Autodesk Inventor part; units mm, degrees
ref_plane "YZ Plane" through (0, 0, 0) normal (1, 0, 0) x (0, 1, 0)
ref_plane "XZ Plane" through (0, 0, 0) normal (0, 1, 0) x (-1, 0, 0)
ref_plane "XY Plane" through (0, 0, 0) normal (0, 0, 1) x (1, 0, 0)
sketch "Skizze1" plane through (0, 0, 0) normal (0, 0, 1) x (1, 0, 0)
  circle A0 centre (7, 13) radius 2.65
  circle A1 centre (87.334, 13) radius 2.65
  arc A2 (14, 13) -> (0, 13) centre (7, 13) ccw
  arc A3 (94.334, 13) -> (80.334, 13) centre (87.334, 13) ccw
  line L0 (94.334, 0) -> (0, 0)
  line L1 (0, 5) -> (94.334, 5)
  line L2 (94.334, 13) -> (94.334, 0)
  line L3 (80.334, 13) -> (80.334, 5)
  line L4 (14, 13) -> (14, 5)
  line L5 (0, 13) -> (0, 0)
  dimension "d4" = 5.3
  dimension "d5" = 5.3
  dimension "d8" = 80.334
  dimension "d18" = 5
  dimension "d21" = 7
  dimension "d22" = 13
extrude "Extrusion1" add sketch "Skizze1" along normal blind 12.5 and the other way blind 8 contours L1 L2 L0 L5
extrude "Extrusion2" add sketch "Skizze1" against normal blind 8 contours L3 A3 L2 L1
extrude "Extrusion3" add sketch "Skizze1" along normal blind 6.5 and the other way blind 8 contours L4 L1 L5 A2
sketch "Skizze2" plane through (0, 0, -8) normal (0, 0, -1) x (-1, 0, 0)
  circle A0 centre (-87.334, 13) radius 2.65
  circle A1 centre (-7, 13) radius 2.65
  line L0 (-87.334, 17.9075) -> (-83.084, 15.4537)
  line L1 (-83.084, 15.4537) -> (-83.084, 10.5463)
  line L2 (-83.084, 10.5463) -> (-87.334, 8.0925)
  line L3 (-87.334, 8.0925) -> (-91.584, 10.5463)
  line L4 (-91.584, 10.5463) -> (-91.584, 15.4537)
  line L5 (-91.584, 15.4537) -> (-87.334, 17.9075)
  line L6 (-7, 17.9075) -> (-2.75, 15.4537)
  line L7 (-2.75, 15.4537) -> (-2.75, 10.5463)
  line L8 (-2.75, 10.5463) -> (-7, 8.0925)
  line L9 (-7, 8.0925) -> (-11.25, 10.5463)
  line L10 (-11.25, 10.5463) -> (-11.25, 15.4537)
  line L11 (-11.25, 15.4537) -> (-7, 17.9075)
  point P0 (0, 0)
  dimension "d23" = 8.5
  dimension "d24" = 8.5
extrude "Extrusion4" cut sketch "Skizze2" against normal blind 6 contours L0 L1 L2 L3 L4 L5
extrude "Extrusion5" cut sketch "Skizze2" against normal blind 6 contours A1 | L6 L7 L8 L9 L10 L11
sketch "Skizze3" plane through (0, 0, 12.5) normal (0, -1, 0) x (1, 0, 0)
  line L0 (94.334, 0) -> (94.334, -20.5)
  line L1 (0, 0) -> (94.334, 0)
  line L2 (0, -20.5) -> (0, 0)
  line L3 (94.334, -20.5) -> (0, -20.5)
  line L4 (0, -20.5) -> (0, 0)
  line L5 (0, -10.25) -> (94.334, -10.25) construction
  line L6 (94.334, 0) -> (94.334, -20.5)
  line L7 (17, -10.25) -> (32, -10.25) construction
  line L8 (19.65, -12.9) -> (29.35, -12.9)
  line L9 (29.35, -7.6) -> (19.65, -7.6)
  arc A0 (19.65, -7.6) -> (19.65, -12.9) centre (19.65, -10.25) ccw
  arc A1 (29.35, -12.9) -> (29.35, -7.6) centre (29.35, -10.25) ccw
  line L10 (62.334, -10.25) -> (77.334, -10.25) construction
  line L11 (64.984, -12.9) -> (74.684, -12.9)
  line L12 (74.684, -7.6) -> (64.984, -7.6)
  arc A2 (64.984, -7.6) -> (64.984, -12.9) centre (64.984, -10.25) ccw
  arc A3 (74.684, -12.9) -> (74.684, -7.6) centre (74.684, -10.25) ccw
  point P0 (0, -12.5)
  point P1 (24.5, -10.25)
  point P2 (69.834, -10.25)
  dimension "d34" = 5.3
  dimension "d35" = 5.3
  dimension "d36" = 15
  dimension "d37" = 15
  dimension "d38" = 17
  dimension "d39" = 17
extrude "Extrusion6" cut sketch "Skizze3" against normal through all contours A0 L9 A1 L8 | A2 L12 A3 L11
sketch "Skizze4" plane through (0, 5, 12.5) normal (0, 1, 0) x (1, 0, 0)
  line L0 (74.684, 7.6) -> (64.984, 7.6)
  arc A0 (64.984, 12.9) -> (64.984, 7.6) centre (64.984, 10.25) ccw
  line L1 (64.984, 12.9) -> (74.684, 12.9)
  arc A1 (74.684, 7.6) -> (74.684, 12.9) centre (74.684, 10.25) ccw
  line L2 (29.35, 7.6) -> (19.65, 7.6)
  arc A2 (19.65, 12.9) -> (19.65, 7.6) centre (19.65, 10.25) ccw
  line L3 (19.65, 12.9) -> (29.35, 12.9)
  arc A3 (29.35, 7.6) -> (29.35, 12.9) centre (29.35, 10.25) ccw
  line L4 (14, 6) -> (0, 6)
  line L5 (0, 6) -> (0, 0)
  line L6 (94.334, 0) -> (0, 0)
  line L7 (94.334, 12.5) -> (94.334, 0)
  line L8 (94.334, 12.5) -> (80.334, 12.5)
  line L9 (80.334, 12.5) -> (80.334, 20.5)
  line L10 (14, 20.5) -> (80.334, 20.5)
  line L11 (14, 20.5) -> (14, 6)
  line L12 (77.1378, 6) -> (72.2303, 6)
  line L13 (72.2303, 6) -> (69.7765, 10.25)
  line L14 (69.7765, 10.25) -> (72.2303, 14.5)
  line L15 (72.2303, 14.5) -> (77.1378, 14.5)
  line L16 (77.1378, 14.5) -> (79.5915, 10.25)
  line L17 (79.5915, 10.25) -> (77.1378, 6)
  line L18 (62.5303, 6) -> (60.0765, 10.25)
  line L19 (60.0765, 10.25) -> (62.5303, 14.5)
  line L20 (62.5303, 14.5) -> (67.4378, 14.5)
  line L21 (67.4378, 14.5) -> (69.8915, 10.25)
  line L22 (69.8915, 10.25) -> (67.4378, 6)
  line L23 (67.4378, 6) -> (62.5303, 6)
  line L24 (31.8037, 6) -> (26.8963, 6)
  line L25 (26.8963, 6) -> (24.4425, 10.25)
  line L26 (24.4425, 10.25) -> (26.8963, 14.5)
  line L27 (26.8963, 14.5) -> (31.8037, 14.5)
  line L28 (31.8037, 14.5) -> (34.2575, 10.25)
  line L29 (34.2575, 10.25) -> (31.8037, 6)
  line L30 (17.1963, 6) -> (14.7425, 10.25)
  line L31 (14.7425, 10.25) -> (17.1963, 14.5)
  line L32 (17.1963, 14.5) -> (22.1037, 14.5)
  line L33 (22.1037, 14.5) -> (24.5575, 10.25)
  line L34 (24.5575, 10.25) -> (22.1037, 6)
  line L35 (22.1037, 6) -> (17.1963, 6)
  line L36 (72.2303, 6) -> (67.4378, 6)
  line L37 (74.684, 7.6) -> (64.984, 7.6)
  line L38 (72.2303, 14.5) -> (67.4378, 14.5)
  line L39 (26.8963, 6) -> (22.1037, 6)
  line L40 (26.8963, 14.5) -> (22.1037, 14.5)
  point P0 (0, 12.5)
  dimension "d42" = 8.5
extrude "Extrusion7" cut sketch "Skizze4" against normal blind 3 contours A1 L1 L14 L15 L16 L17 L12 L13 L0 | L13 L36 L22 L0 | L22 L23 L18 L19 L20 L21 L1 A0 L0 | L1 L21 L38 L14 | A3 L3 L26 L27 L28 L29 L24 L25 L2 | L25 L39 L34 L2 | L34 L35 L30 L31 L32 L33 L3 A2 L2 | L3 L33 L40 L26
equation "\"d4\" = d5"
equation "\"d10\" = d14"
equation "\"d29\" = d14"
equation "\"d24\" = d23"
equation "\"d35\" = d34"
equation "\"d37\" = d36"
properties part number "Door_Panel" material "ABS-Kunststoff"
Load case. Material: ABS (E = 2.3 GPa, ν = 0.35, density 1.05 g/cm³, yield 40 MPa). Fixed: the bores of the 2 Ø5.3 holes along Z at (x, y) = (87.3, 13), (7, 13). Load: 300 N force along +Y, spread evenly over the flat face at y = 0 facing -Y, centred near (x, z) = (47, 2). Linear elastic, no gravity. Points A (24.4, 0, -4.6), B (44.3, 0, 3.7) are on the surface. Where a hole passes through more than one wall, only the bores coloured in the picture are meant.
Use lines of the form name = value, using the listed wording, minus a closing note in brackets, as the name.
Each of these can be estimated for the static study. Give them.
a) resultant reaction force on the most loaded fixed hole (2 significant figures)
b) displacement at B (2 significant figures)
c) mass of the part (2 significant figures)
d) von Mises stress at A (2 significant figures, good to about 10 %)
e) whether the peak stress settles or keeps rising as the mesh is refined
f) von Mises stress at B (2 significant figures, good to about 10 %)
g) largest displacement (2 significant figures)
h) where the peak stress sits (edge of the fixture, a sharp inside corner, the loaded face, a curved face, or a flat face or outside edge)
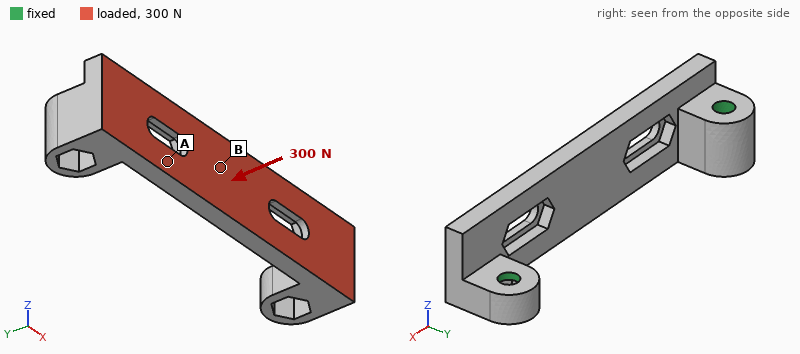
resultant reaction force on the most loaded fixed hole = 180 N
displacement at B = 0.73 mm
mass of the part = 12 g
von Mises stress at A = 2.6 MPa
whether the peak stress settles or keeps rising as the mesh is refined = keeps rising
von Mises stress at B = 9.9 MPa
largest displacement = 0.89 mm
where the peak stress sits = edge of the fixture
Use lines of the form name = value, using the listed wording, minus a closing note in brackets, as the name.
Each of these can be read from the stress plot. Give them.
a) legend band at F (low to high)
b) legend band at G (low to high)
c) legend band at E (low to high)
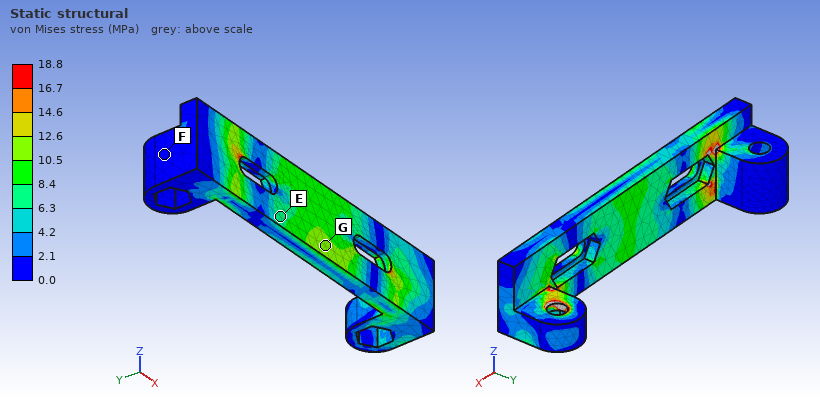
legend band at F = 0.0 to 2.1 MPa
legend band at G = 10.5 to 12.6 MPa
legend band at E = 6.3 to 8.4 MPa
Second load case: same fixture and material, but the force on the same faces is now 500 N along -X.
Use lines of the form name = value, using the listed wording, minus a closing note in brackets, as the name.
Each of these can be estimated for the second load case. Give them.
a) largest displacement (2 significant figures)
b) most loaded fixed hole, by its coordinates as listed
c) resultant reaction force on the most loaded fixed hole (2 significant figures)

largest displacement = 0.18 mm
most loaded fixed hole, by its coordinates as listed = (7, 13)
resultant reaction force on the most loaded fixed hole = 350 N
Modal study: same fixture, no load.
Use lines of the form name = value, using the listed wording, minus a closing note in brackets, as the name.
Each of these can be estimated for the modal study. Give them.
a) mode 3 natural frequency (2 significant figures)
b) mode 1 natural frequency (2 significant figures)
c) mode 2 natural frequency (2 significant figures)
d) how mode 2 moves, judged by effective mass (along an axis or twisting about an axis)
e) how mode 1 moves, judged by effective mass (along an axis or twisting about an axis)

mode 3 natural frequency = 2100 Hz
mode 1 natural frequency = 1200 Hz
mode 2 natural frequency = 1500 Hz
how mode 2 moves, judged by effective mass = along Z
how mode 1 moves, judged by effective mass = along Y
